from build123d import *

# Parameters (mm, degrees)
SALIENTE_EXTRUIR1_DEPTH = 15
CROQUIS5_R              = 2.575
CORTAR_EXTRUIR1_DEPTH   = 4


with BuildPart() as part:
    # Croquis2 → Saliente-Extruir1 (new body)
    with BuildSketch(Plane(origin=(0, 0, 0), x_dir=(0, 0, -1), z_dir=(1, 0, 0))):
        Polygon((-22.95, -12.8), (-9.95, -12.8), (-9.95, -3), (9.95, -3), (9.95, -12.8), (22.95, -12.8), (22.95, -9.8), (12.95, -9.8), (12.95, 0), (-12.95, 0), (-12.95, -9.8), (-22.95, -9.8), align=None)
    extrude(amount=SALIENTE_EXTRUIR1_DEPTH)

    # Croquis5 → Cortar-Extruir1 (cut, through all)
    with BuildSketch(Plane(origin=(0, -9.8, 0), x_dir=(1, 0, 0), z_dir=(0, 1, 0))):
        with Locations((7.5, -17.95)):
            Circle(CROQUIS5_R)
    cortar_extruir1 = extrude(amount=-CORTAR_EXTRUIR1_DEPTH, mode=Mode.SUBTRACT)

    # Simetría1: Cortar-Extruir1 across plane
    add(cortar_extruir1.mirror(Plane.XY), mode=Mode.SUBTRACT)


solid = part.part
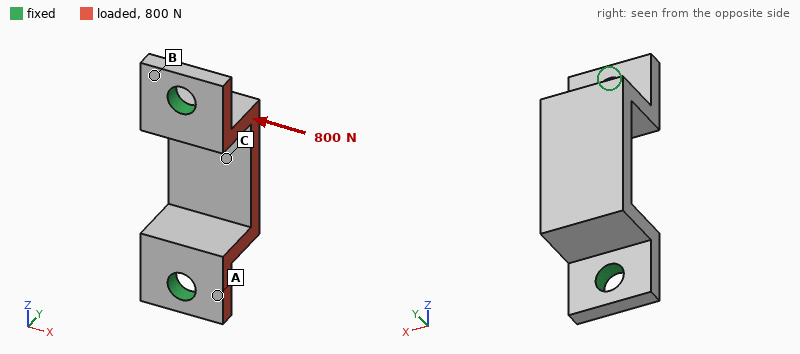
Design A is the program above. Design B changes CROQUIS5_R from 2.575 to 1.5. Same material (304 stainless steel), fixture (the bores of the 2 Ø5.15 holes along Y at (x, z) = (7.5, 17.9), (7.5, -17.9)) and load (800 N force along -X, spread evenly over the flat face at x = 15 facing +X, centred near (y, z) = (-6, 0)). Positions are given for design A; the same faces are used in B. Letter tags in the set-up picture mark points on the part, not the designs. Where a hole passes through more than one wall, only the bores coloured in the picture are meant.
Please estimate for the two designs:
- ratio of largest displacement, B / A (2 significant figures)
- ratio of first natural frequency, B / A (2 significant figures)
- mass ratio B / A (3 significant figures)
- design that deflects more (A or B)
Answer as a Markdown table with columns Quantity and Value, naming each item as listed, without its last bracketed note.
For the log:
| Quantity | Value |
|---|---|
| ratio of largest displacement, B / A | 1.7 |
| ratio of first natural frequency, B / A | 0.77 |
| mass ratio B / A | 1.03 |
| design that deflects more | B |
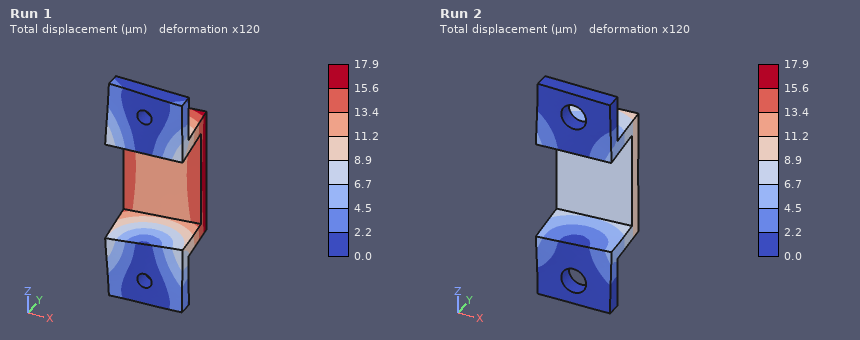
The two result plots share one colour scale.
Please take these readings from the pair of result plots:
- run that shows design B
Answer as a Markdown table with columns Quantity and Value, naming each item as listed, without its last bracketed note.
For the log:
| Quantity | Value |
|---|---|
| run that shows design B | Run 1 |
